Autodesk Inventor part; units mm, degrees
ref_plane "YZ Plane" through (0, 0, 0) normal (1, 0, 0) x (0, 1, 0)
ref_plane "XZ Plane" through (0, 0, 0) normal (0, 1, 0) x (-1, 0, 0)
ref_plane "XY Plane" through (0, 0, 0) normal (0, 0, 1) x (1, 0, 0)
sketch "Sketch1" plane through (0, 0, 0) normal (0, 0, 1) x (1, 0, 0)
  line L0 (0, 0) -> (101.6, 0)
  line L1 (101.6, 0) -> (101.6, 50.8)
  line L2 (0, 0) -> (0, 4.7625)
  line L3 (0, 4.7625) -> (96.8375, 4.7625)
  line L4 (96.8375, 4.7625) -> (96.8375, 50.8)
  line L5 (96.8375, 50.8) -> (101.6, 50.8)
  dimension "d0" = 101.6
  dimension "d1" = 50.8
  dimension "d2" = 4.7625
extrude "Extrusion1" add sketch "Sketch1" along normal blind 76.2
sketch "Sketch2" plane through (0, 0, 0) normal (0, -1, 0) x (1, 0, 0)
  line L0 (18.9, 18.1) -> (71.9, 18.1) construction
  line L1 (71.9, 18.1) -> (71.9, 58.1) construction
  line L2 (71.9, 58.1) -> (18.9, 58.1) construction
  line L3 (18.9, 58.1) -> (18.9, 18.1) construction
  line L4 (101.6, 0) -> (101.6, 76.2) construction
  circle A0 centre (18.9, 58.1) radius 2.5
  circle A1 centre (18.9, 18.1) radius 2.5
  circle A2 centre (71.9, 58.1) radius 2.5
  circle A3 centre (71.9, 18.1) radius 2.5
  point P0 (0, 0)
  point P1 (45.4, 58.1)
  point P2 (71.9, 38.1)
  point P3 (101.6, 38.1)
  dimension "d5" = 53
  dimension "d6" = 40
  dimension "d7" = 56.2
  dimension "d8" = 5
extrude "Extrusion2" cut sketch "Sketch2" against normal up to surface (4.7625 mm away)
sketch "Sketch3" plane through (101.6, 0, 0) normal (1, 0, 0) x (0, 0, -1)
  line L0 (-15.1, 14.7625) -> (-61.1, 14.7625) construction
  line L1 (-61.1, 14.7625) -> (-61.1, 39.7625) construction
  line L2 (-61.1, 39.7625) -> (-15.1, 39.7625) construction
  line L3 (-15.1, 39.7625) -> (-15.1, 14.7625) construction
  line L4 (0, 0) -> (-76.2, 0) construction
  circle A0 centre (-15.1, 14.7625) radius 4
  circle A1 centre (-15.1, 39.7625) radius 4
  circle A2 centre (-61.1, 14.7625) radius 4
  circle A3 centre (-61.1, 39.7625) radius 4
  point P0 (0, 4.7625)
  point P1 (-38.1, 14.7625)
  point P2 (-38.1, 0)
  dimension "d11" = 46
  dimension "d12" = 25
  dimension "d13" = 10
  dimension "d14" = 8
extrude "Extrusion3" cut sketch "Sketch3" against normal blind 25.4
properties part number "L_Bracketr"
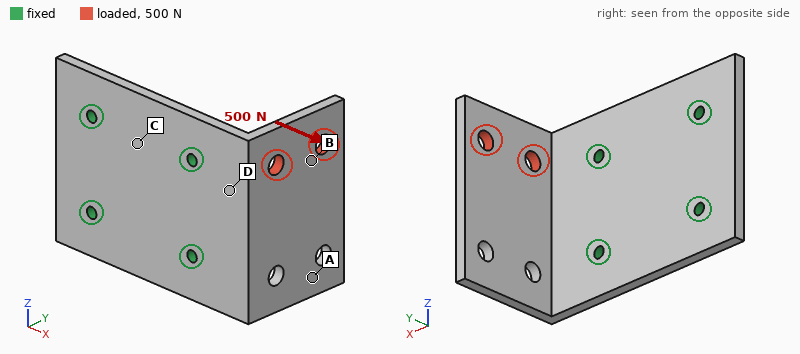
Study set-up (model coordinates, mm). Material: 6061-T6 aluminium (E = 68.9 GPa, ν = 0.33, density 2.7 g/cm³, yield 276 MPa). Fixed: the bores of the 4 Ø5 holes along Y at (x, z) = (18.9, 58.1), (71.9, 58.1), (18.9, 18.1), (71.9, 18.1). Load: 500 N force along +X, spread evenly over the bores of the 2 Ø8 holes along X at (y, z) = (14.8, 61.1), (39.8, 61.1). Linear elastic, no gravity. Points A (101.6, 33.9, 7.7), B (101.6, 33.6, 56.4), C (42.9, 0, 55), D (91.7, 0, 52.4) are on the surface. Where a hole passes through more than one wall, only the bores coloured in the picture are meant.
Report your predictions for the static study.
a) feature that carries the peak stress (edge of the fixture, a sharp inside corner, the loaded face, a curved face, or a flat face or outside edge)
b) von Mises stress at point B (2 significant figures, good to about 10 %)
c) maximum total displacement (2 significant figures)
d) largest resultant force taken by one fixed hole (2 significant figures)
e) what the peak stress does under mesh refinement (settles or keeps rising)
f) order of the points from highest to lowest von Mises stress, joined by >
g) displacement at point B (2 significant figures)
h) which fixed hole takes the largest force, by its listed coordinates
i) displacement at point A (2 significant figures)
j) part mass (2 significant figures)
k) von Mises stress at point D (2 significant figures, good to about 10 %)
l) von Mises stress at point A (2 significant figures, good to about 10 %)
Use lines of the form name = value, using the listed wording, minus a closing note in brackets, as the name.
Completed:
feature that carries the peak stress = edge of the fixture
von Mises stress at point B = 20 MPa
maximum total displacement = 0.62 mm
largest resultant force taken by one fixed hole = 410 N
what the peak stress does under mesh refinement = keeps rising
order of the points from highest to lowest von Mises stress, joined by > = D > B > A > C
displacement at point B = 0.37 mm
which fixed hole takes the largest force, by its listed coordinates = (71.9, 58.1)
displacement at point A = 0.24 mm
part mass = 140 g
von Mises stress at point D = 45 MPa
von Mises stress at point A = 12 MPa
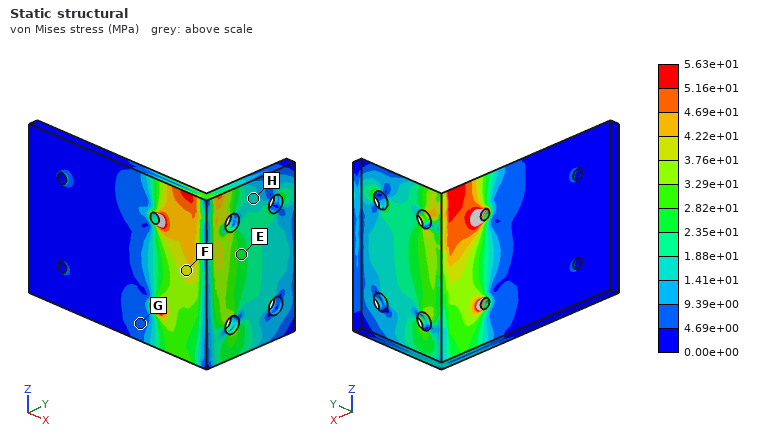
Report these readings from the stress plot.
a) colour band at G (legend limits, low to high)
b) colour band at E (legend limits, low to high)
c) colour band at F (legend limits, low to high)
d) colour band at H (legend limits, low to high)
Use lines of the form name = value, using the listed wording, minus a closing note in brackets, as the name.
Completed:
colour band at G = 4.69e+00 to 9.39e+00 MPa
colour band at E = 2.35e+01 to 2.82e+01 MPa
colour band at F = 3.76e+01 to 4.22e+01 MPa
colour band at H = 1.41e+01 to 1.88e+01 MPa
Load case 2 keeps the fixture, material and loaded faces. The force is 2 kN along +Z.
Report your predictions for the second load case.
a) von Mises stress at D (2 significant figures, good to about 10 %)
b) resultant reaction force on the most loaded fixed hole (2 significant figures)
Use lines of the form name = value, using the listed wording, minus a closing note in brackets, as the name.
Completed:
von Mises stress at D = 50 MPa
resultant reaction force on the most loaded fixed hole = 1.8 kN
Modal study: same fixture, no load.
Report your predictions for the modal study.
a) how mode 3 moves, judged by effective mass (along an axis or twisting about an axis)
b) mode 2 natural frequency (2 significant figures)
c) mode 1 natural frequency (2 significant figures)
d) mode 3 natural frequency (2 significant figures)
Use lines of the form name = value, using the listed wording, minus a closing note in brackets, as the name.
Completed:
how mode 3 moves, judged by effective mass = along Y
mode 2 natural frequency = 1600 Hz
mode 1 natural frequency = 880 Hz
mode 3 natural frequency = 2700 Hz
